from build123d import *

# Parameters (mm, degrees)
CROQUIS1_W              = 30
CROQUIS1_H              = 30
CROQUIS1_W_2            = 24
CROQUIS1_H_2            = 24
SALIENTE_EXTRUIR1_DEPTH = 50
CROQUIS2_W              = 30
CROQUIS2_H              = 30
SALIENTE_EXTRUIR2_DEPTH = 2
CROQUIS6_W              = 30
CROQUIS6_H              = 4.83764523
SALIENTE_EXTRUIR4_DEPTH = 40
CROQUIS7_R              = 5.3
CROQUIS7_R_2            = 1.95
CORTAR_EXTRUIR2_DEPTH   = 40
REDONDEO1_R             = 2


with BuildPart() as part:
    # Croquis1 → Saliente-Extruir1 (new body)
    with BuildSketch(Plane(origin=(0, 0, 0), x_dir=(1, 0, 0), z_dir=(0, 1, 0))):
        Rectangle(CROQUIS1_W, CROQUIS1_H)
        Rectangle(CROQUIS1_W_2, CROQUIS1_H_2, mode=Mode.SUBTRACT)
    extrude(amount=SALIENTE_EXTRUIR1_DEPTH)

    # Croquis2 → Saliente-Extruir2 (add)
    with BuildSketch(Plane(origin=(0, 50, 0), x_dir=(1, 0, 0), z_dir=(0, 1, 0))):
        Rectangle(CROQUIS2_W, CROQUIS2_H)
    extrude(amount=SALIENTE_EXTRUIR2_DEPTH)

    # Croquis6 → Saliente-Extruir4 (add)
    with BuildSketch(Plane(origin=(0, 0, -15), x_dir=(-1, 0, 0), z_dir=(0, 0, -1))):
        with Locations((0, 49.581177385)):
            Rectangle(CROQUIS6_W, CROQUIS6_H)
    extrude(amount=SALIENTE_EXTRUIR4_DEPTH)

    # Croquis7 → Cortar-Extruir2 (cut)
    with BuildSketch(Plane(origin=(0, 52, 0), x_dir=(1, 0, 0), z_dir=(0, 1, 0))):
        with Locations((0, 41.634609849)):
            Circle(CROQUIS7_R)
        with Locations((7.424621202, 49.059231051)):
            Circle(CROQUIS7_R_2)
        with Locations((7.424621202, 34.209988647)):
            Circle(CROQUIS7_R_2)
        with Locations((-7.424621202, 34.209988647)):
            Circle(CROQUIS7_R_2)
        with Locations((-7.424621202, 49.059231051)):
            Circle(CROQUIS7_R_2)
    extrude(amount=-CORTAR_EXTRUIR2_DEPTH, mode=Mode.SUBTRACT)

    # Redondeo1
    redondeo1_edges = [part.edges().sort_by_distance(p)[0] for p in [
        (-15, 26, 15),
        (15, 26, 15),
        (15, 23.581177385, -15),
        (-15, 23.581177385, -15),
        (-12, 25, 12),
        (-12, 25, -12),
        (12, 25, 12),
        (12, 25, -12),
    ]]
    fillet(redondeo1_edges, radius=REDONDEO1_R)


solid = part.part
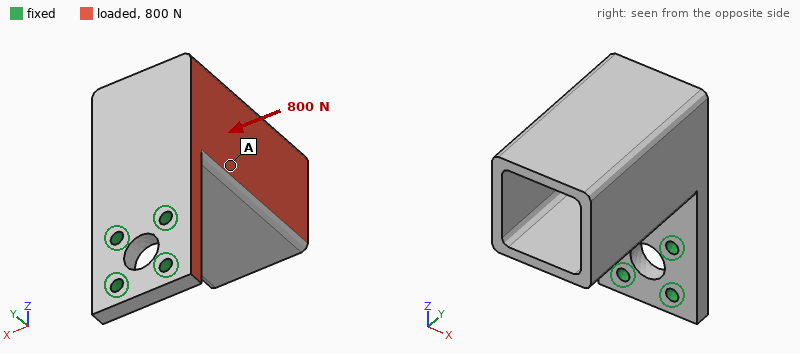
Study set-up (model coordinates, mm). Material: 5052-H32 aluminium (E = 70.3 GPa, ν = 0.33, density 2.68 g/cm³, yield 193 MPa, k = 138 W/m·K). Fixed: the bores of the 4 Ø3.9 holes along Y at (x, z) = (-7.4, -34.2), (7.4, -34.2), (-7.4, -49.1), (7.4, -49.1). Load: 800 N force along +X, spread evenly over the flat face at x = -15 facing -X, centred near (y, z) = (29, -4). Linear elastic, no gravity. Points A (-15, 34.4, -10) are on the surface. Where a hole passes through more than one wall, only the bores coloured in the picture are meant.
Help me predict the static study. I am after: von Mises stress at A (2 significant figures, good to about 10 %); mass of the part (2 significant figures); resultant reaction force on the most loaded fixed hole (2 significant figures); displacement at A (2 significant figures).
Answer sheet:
14 MPa
62 g
1.5 kN
0.15 mm
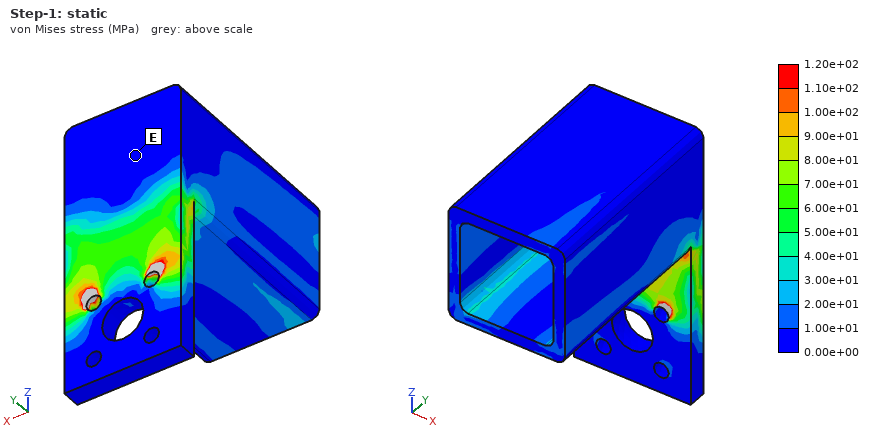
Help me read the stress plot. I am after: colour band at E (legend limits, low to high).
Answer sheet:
0.00e+00 to 1.00e+01 MPa
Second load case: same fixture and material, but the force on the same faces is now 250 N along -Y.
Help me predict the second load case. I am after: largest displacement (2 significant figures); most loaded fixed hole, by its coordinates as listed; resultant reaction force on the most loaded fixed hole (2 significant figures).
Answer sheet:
0.38 mm
(-7.4, -34.2)
340 N
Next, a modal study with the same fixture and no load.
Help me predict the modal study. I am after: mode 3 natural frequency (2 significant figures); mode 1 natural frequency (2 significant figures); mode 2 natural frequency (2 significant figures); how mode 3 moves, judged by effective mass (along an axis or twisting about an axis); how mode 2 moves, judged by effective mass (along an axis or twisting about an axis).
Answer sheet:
3600 Hz
570 Hz
1200 Hz
along Y
along X
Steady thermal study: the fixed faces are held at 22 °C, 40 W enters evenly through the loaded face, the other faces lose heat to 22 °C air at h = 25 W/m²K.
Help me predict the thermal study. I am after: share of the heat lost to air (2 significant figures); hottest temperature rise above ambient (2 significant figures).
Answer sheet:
29 %
55 K
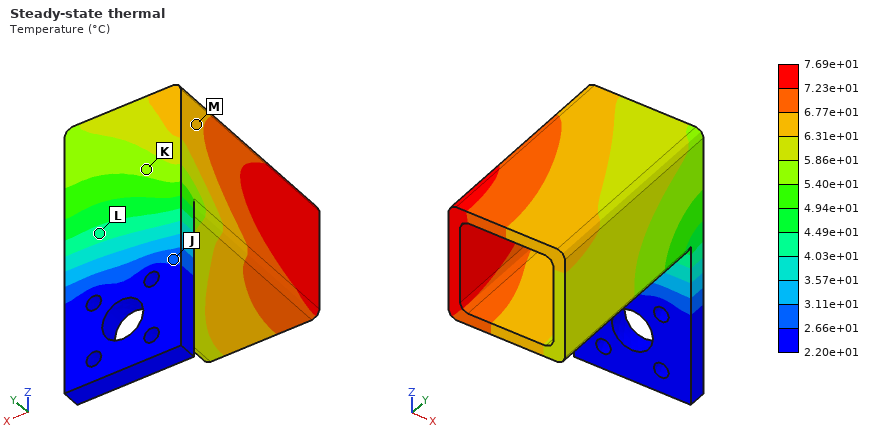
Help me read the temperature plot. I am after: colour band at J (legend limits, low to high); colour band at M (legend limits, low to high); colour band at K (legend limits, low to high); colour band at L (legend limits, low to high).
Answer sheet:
2.66e+01 to 3.11e+01 °C
6.31e+01 to 6.77e+01 °C
5.40e+01 to 5.86e+01 °C
4.03e+01 to 4.49e+01 °C
